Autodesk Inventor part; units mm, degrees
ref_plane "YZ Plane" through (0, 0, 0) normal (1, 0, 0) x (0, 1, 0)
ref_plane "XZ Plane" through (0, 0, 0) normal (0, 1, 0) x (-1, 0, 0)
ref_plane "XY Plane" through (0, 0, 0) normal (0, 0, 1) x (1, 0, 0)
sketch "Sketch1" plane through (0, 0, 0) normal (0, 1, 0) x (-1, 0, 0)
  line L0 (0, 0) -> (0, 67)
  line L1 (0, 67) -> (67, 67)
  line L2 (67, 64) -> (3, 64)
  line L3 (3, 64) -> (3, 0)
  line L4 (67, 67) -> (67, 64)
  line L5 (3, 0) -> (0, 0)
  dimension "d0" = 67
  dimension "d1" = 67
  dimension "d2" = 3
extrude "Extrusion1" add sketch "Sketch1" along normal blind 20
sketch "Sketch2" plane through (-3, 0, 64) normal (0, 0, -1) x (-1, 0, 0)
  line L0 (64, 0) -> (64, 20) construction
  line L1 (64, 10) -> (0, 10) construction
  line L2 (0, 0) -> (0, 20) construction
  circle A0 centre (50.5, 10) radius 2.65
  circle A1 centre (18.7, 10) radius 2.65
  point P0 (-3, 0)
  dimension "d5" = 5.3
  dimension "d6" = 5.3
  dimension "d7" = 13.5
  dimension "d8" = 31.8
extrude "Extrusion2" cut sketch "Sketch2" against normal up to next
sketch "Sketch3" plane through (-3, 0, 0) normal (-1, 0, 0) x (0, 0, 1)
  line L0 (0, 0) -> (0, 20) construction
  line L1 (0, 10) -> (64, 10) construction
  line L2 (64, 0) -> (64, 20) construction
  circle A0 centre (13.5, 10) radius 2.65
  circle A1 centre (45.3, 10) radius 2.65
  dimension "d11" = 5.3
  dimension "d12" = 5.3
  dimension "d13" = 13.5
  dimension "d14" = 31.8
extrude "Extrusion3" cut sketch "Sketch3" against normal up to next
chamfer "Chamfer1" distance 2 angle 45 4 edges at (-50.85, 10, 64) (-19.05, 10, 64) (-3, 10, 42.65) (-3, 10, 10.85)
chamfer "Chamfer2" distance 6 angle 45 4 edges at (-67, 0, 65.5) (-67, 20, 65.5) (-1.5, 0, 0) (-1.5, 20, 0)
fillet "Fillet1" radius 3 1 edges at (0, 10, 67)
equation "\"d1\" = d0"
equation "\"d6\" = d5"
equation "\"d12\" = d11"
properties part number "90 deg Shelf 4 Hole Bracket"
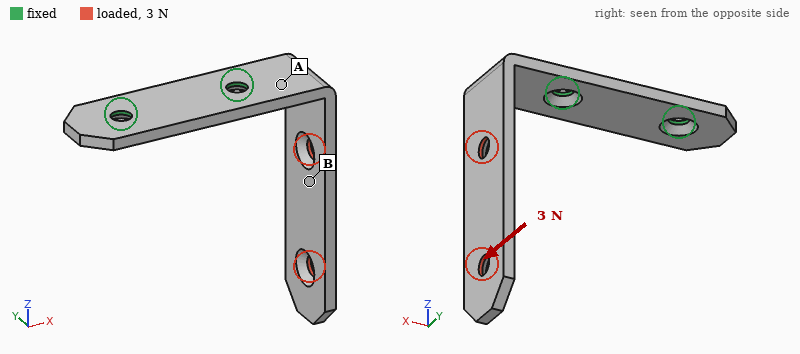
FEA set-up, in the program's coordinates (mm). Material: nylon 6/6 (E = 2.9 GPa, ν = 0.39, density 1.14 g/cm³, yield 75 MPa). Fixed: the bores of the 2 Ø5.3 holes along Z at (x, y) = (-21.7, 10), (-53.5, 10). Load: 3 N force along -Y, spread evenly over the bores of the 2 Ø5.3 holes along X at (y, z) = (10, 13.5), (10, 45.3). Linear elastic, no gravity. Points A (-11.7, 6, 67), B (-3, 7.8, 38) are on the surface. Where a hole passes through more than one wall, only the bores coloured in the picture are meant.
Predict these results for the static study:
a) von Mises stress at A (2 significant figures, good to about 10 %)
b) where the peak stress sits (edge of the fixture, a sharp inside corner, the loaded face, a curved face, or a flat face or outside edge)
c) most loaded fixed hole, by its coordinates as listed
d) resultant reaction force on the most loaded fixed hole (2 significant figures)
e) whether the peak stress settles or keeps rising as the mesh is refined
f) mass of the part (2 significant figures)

2.9 MPa
edge of the fixture
(-21.7, 10)
3.6 N
keeps rising
8.2 g
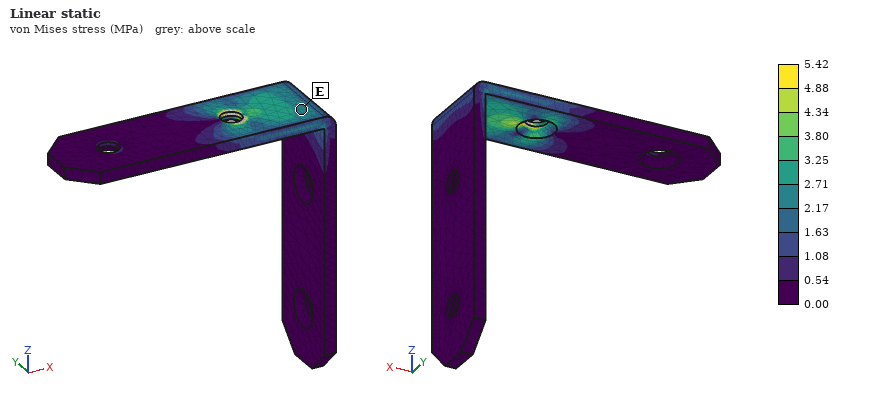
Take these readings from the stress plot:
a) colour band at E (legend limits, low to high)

2.17 to 2.71 MPa
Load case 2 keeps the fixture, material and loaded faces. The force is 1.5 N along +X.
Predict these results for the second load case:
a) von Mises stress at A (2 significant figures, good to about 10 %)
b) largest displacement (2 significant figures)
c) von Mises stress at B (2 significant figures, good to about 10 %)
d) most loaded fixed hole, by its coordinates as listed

1.6 MPa
1.1 mm
0.53 MPa
(-53.5, 10)
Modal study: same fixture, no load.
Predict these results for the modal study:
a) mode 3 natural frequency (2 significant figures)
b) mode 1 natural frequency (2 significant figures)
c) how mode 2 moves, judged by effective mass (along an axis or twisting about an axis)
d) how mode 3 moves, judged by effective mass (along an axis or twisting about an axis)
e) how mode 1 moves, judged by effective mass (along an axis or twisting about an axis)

570 Hz
120 Hz
along Y
along Z
along X
